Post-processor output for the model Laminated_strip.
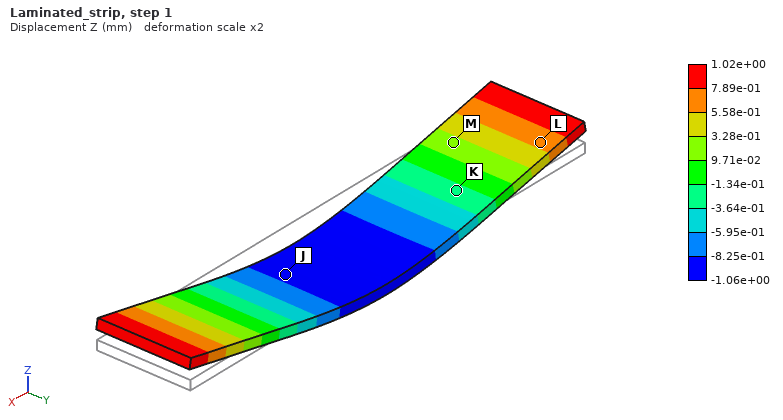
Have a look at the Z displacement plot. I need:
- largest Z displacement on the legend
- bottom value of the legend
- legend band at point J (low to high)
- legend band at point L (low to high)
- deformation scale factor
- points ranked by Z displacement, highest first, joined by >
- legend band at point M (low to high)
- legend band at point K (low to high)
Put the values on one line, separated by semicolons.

1.02e+00 mm; -1.06e+00 mm; -1.06e+00 to -8.25e-01 mm; 5.58e-01 to 7.89e-01 mm; 2; L > M > K > J; 9.71e-02 to 3.28e-01 mm; -3.64e-01 to -1.34e-01 mm
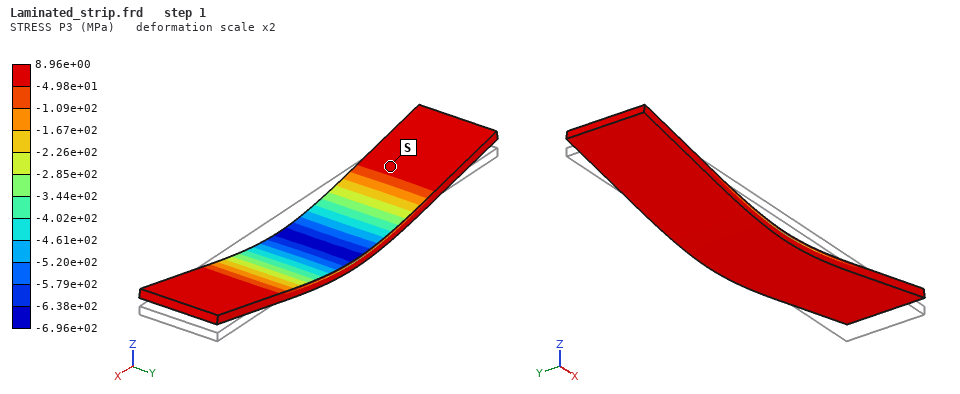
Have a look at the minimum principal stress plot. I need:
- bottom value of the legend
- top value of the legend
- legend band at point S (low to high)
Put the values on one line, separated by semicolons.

-6.96e+02 MPa; 8.96e+00 MPa; -4.98e+01 to 8.96e+00 MPa
